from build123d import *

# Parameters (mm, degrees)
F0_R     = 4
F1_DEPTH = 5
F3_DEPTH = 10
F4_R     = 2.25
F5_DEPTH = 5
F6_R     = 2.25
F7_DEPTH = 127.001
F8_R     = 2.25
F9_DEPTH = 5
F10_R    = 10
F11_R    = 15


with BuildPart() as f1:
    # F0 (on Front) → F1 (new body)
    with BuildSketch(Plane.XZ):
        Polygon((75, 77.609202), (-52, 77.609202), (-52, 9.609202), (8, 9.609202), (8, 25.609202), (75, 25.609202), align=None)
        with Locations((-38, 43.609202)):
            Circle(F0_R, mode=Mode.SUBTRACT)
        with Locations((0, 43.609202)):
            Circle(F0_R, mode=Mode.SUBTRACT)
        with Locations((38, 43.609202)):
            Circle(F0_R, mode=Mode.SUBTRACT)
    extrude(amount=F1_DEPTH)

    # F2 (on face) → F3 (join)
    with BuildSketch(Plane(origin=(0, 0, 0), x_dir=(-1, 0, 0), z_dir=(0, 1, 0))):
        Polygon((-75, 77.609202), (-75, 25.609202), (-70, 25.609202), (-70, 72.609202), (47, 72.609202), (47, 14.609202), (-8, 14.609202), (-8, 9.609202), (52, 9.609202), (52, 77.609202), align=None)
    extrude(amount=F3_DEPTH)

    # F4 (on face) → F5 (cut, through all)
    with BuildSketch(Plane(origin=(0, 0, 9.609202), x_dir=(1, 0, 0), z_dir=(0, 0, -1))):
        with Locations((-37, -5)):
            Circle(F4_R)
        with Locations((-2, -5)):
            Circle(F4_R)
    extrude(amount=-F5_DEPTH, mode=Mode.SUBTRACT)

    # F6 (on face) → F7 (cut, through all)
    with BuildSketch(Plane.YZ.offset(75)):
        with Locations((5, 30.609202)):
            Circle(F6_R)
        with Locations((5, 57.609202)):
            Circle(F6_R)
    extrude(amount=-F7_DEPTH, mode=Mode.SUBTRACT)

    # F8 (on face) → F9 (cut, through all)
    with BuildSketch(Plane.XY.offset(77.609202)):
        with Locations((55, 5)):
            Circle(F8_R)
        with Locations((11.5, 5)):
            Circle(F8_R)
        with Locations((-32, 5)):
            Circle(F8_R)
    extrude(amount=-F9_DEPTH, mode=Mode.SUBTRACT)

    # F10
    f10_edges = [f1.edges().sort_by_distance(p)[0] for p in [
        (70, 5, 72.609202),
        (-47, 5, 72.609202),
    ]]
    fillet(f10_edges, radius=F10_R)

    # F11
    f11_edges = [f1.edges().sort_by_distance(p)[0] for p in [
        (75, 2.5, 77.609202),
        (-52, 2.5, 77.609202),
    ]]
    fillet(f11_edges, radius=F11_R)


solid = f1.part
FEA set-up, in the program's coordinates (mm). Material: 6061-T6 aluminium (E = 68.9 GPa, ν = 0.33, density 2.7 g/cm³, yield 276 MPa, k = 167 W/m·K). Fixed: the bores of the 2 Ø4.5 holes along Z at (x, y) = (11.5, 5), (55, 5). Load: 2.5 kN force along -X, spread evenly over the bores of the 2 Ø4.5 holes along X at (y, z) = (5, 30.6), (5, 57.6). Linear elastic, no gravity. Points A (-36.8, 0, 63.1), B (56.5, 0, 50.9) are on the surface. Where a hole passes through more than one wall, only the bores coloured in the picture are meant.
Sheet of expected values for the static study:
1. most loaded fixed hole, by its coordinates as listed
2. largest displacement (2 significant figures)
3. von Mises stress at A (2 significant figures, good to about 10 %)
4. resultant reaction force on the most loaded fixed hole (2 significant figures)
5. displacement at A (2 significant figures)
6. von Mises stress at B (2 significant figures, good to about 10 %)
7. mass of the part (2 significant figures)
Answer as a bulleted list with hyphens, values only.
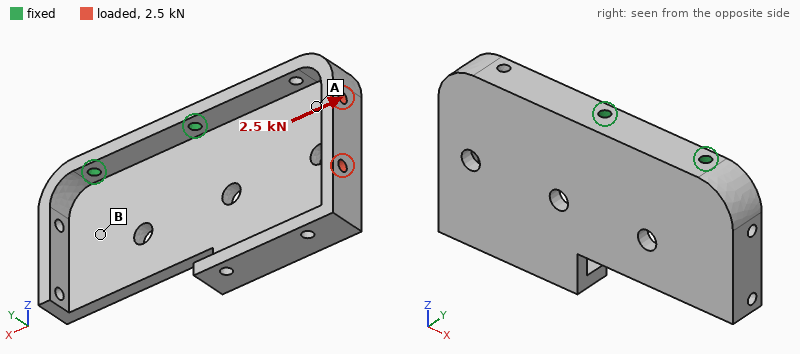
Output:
- (11.5, 5)
- 0.59 mm
- 33 MPa
- 2.5 kN
- 0.20 mm
- 15 MPa
- 130 g
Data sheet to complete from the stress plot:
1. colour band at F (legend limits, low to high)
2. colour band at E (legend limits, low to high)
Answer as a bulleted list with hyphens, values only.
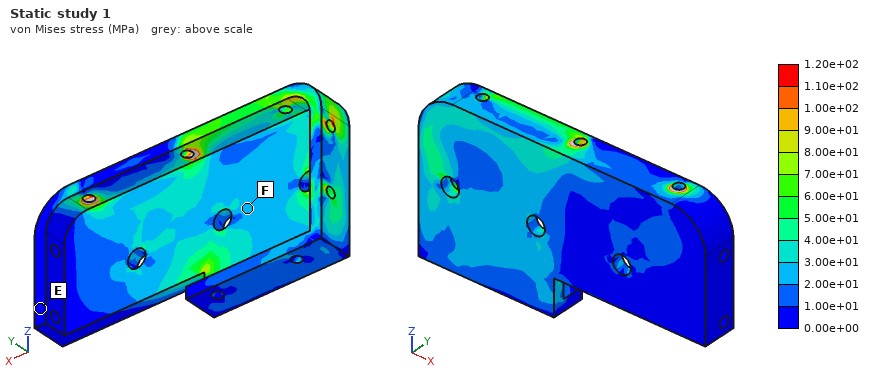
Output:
- 2.00e+01 to 3.00e+01 MPa
- 0.00e+00 to 1.00e+01 MPa
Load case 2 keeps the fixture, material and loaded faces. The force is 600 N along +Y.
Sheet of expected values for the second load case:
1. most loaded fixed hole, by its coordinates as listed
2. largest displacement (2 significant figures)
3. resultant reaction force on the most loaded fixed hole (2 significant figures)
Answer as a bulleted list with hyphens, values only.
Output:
- (11.5, 5)
- 1.5 mm
- 1.6 kN
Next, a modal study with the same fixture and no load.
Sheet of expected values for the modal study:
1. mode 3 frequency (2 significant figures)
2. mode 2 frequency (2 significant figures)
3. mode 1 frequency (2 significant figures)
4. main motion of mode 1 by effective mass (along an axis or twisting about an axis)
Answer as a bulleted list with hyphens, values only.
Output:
- 2000 Hz
- 1400 Hz
- 530 Hz
- along Y
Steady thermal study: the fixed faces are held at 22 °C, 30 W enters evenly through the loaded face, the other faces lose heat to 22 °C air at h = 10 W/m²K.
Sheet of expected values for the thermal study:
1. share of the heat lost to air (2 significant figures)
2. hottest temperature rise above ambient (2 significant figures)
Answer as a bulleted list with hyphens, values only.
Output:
- 14 %
- 48 K
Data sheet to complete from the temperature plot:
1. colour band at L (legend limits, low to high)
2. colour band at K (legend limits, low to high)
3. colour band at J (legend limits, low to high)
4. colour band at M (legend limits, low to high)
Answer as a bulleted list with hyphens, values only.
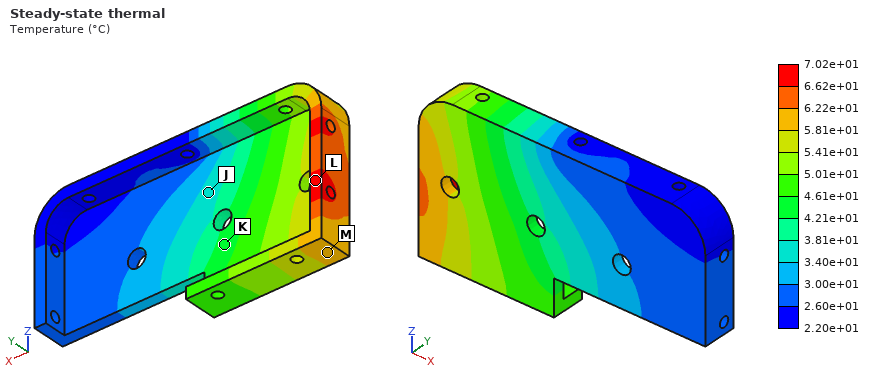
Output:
- 6.62e+01 to 7.02e+01 °C
- 4.21e+01 to 4.61e+01 °C
- 3.40e+01 to 3.81e+01 °C
- 5.81e+01 to 6.22e+01 °C
